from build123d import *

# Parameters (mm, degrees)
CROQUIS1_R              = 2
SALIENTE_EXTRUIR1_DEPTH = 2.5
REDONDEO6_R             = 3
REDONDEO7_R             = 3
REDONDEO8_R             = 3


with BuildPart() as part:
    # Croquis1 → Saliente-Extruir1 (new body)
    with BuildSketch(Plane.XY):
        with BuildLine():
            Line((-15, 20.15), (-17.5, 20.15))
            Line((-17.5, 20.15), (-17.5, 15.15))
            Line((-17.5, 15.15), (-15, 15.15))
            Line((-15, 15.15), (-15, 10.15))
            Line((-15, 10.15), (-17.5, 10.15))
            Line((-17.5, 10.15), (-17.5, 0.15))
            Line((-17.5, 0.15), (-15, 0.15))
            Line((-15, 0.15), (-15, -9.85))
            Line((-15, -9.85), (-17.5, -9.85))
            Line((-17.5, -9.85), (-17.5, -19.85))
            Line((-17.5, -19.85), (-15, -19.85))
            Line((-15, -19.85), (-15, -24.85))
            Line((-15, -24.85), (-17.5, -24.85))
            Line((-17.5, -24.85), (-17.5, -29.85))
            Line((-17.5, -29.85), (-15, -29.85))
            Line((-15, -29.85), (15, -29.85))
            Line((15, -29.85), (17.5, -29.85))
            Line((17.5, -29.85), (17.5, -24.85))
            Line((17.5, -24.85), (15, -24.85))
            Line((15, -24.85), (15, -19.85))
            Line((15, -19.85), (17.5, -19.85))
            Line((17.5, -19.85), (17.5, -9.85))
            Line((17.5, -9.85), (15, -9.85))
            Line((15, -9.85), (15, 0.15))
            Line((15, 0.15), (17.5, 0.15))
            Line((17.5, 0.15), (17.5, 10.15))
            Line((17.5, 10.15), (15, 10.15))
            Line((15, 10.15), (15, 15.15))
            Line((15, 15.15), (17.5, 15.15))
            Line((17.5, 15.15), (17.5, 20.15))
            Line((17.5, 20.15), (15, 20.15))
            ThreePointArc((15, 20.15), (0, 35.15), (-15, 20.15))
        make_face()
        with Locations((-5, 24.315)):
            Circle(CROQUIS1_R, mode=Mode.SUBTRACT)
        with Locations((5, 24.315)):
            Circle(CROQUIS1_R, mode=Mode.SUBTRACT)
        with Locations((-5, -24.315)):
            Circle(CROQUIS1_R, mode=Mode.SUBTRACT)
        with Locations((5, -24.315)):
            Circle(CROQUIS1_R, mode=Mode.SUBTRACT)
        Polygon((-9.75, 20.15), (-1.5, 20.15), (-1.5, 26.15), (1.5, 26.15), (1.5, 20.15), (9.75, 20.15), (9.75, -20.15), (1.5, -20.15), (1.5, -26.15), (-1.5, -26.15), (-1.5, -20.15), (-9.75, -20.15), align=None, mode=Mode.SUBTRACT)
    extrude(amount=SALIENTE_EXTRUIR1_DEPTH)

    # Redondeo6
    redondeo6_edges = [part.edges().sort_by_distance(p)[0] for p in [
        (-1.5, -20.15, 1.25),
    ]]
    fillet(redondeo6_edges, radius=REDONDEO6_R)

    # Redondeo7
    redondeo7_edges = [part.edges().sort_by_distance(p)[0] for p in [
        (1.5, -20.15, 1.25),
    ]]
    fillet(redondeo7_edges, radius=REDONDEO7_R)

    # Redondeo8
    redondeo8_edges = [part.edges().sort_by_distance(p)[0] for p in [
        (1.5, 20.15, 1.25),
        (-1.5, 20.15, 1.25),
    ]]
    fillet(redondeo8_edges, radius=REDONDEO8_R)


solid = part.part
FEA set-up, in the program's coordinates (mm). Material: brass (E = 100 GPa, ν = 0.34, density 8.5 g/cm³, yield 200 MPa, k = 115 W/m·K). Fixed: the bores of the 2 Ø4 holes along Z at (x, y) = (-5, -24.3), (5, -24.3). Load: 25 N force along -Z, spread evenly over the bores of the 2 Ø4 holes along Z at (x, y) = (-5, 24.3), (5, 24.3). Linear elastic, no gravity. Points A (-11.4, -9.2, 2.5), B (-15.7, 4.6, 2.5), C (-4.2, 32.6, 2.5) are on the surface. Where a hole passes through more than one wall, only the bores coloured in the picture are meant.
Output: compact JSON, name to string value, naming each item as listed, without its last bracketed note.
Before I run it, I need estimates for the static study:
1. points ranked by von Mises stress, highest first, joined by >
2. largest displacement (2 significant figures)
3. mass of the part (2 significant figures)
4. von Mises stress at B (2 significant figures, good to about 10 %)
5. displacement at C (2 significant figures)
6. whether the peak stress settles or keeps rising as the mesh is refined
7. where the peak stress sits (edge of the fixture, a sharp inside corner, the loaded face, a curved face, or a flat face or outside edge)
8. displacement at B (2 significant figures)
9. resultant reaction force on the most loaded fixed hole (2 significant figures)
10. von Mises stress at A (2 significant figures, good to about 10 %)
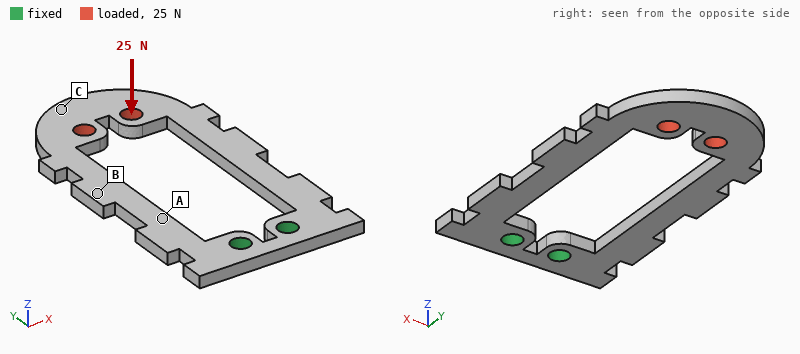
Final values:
{"points ranked by von Mises stress, highest first, joined by >": "A > B > C", "largest displacement": "0.86 mm", "mass of the part": "24 g", "von Mises stress at B": "27 MPa", "displacement at C": "0.81 mm", "whether the peak stress settles or keeps rising as the mesh is refined": "keeps rising", "where the peak stress sits": "a sharp inside corner", "displacement at B": "0.28 mm", "resultant reaction force on the most loaded fixed hole": "13 N", "von Mises stress at A": "72 MPa"}
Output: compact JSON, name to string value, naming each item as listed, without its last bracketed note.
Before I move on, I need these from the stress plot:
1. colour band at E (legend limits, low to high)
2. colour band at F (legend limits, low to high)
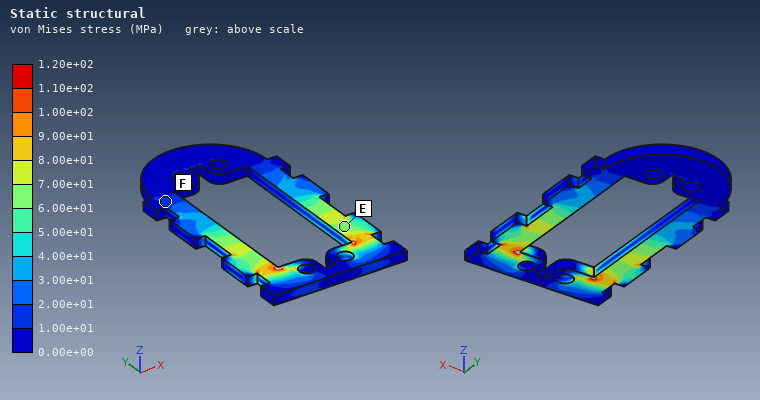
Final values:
{"colour band at E": "6.00e+01 to 7.00e+01 MPa", "colour band at F": "1.00e+01 to 2.00e+01 MPa"}
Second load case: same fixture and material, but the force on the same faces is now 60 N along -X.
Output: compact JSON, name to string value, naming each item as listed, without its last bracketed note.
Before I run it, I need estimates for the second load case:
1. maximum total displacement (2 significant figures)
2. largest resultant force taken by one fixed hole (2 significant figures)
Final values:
{"maximum total displacement": "96 µm", "largest resultant force taken by one fixed hole": "98 N"}
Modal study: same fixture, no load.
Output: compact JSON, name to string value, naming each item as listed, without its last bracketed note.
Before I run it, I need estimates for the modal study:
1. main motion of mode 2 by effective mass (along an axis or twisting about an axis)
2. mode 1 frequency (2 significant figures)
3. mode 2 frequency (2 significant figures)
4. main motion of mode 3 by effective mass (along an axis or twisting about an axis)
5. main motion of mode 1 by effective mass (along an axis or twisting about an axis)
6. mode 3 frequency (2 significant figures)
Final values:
{"main motion of mode 2 by effective mass": "twisting about Y", "mode 1 frequency": "310 Hz", "mode 2 frequency": "1000 Hz", "main motion of mode 3 by effective mass": "along X", "main motion of mode 1 by effective mass": "along Z", "mode 3 frequency": "1200 Hz"}
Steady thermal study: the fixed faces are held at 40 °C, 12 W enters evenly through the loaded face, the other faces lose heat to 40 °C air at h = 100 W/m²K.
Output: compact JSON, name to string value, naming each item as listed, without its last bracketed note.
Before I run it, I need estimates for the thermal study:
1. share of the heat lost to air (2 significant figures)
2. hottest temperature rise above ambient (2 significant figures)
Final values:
{"share of the heat lost to air": "77 %", "hottest temperature rise above ambient": "73 K"}
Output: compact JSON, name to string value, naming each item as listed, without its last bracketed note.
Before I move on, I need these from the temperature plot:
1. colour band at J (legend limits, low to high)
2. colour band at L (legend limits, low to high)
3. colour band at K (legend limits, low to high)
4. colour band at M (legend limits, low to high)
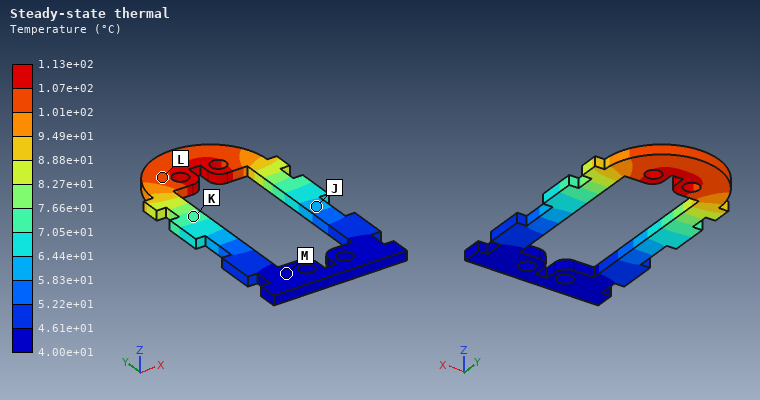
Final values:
{"colour band at J": "5.83e+01 to 6.44e+01 °C", "colour band at L": "1.01e+02 to 1.07e+02 °C", "colour band at K": "7.05e+01 to 7.66e+01 °C", "colour band at M": "4.00e+01 to 4.61e+01 °C"}
